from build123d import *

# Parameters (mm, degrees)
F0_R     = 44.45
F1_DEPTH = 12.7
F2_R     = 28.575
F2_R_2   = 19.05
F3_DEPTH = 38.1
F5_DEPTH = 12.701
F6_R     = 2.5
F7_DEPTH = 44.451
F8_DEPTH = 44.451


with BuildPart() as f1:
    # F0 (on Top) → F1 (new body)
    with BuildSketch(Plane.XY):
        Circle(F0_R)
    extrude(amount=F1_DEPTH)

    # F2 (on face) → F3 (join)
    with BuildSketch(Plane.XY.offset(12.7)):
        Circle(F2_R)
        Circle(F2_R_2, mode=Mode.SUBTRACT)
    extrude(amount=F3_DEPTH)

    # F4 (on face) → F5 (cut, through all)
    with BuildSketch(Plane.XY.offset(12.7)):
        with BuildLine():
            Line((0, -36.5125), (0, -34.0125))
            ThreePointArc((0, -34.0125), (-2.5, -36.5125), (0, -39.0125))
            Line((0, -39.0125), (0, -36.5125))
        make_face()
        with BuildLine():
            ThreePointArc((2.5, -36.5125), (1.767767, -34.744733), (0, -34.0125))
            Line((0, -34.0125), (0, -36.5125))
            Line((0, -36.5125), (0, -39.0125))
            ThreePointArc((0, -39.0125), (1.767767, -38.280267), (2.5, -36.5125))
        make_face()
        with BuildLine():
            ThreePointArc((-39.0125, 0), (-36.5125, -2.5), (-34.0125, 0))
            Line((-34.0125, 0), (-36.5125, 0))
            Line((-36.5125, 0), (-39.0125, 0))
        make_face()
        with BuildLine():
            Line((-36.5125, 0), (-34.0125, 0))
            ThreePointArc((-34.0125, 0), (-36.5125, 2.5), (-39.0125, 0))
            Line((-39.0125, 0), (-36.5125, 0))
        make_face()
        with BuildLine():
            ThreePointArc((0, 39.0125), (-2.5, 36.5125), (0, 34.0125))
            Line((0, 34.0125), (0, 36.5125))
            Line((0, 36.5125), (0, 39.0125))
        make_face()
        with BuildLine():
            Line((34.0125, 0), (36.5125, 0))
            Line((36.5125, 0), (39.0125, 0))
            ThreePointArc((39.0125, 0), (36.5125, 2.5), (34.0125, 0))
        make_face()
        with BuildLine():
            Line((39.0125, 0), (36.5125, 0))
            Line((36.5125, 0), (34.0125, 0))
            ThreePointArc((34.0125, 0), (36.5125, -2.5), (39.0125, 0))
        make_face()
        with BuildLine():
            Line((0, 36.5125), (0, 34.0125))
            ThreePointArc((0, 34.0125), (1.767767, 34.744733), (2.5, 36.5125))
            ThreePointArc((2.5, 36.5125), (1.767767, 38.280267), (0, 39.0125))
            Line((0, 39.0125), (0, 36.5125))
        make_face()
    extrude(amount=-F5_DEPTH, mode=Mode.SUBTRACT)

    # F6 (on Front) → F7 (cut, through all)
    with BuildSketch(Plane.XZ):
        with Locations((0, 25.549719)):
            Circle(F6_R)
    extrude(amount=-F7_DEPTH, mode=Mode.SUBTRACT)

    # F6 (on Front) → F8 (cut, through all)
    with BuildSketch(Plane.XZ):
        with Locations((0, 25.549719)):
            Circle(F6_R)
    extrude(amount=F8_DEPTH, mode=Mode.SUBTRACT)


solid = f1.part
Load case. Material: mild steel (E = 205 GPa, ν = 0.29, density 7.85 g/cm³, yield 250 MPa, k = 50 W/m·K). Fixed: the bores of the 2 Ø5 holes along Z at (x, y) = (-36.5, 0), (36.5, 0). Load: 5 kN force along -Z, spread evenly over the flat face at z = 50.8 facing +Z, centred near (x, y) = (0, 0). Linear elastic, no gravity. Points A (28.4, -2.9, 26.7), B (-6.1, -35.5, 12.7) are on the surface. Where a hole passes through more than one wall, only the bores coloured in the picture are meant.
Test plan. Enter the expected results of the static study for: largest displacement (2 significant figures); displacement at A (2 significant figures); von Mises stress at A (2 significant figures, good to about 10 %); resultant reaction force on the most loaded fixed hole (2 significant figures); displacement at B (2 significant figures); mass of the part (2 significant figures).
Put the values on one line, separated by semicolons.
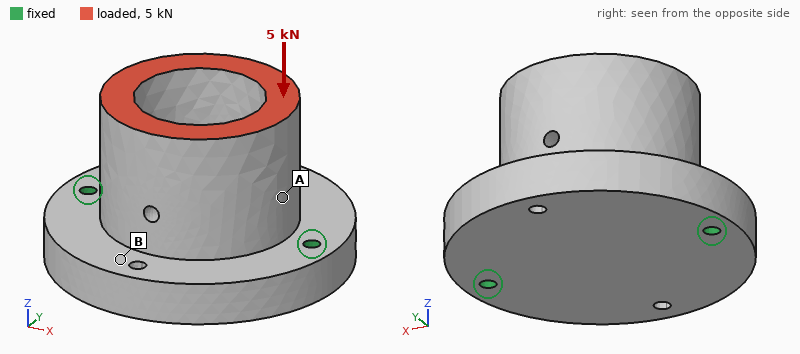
4.6 µm; 2.9 µm; 7.0 MPa; 2.6 kN; 4.1 µm; 1.0 kg
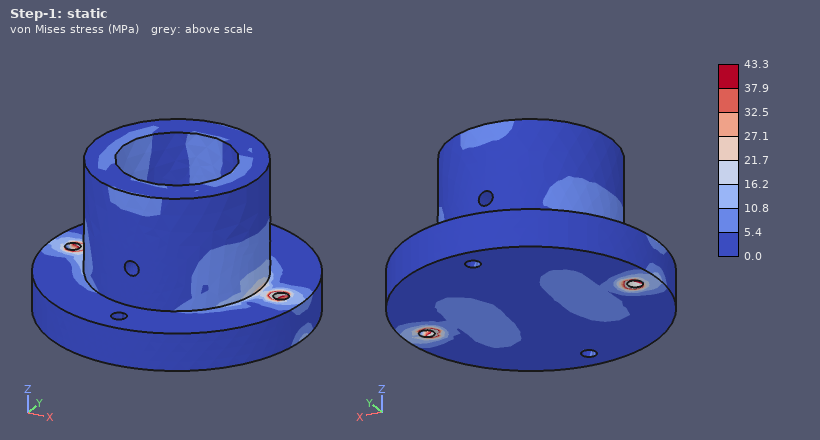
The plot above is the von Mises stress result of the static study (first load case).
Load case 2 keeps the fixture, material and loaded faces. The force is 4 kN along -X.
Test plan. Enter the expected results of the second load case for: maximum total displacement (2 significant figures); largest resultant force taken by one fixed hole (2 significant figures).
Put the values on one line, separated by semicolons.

8.8 µm; 3.3 kN
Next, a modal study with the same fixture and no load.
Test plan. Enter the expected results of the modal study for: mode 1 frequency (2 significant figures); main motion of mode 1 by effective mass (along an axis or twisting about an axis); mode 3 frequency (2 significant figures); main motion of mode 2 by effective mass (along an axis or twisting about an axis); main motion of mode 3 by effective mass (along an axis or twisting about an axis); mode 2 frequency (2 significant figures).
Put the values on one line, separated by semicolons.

2500 Hz; along Y; 8100 Hz; along Z; along X; 6000 Hz
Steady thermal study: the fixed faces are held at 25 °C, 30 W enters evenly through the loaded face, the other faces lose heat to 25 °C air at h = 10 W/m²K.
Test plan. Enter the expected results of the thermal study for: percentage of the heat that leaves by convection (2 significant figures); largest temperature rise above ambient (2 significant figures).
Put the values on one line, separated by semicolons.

12 %; 27 K
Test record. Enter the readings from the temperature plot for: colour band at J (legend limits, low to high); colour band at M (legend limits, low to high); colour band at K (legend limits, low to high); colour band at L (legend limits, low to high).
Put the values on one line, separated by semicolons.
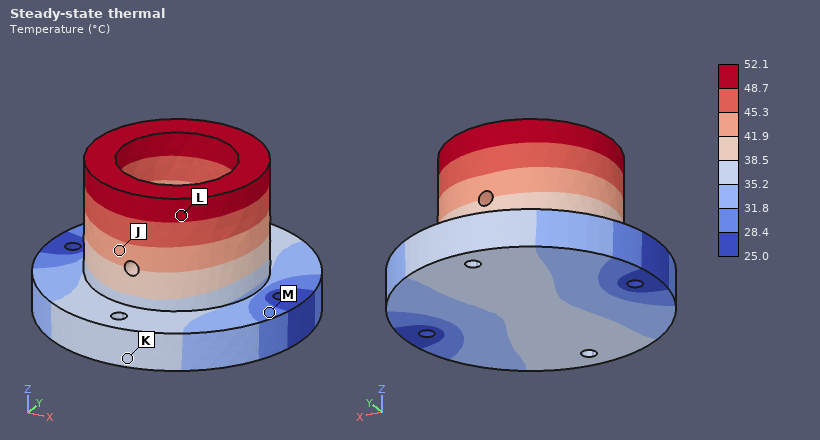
41.9 to 45.3 °C; 28.4 to 31.8 °C; 35.2 to 38.5 °C; 48.7 to 52.1 °C
